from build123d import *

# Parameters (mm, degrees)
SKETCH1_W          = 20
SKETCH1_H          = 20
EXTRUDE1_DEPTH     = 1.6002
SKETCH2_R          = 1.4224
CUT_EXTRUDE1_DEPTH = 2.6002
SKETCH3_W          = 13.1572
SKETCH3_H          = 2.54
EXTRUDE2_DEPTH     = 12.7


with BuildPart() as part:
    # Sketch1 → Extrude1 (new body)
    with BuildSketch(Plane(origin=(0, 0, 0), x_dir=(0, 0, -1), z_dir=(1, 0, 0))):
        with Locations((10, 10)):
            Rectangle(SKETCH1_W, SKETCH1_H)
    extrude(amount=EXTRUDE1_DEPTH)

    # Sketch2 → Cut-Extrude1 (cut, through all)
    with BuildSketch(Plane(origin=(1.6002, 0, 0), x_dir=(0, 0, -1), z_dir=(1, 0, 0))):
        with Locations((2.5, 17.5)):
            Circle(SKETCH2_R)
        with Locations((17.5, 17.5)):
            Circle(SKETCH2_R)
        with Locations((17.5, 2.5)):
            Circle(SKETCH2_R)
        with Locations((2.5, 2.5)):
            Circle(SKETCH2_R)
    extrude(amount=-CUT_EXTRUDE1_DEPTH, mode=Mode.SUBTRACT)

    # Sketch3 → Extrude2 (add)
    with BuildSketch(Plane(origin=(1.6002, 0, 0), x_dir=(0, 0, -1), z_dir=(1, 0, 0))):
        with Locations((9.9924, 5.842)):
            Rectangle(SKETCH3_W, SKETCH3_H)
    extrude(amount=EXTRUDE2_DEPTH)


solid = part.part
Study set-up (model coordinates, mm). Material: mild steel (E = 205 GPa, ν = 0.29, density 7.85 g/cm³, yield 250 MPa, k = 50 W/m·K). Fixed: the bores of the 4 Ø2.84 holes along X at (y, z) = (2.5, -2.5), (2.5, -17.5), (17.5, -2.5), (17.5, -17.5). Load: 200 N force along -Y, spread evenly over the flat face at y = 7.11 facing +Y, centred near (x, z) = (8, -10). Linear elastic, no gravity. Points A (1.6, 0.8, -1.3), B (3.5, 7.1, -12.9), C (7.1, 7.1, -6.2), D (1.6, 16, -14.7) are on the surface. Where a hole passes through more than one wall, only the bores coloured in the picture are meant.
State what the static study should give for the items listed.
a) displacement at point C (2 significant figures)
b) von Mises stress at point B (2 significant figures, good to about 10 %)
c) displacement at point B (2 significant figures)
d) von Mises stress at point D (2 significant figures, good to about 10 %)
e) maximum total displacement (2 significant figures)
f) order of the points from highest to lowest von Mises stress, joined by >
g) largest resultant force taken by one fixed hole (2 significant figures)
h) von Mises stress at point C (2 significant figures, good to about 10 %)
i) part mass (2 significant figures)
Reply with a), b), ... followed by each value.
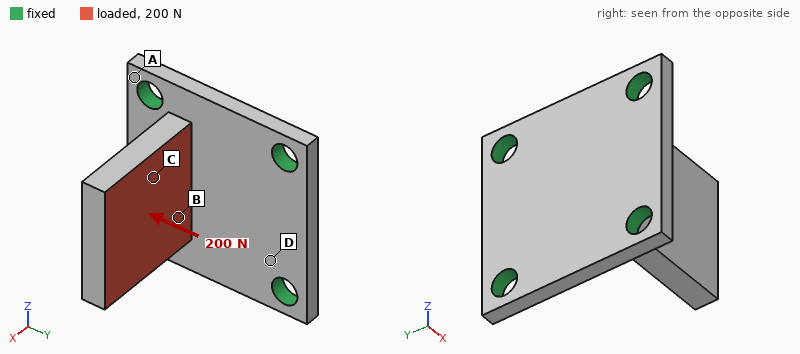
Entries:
a) 13 µm
b) 58 MPa
c) 5.7 µm
d) 19 MPa
e) 32 µm
f) B > C > D > A
g) 87 N
h) 29 MPa
i) 8.0 g
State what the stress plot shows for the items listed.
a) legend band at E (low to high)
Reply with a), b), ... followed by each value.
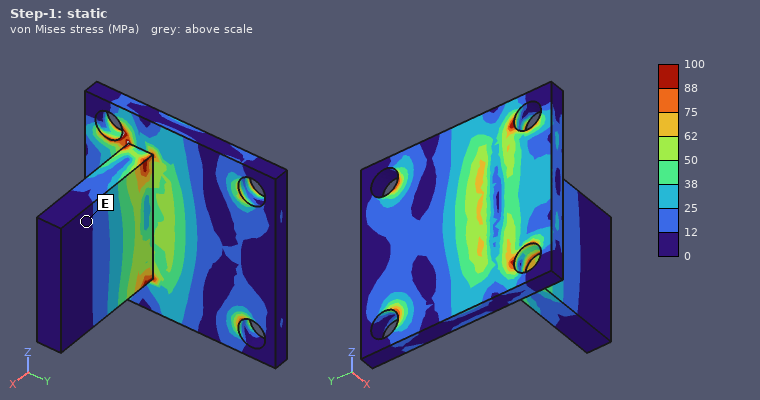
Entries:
a) 0 to 12 MPa
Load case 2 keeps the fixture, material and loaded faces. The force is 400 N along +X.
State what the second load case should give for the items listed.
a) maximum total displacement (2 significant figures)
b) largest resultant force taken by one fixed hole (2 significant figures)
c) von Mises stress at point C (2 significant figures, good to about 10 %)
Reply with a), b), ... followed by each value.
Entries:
a) 20 µm
b) 160 N
c) 27 MPa
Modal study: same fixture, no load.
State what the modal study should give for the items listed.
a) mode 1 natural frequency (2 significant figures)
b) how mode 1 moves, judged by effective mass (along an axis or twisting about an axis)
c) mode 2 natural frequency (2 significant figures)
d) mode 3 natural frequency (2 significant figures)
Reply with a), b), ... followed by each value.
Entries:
a) 8500 Hz
b) along Y
c) 23 kHz
d) 27 kHz
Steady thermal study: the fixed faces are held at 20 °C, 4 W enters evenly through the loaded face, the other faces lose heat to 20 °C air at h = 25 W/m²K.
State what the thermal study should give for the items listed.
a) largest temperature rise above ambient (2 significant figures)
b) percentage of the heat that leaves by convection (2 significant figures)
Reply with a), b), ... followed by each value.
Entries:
a) 24 K
b) 4.9 %
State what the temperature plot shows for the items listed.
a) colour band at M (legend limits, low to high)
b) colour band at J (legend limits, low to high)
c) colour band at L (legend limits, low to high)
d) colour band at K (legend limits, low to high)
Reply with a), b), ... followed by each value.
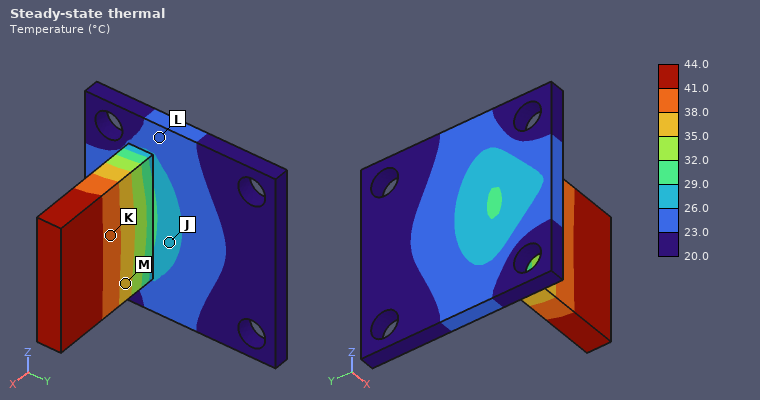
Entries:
a) 35.0 to 38.0 °C
b) 26.0 to 29.0 °C
c) 23.0 to 26.0 °C
d) 38.0 to 41.0 °C
